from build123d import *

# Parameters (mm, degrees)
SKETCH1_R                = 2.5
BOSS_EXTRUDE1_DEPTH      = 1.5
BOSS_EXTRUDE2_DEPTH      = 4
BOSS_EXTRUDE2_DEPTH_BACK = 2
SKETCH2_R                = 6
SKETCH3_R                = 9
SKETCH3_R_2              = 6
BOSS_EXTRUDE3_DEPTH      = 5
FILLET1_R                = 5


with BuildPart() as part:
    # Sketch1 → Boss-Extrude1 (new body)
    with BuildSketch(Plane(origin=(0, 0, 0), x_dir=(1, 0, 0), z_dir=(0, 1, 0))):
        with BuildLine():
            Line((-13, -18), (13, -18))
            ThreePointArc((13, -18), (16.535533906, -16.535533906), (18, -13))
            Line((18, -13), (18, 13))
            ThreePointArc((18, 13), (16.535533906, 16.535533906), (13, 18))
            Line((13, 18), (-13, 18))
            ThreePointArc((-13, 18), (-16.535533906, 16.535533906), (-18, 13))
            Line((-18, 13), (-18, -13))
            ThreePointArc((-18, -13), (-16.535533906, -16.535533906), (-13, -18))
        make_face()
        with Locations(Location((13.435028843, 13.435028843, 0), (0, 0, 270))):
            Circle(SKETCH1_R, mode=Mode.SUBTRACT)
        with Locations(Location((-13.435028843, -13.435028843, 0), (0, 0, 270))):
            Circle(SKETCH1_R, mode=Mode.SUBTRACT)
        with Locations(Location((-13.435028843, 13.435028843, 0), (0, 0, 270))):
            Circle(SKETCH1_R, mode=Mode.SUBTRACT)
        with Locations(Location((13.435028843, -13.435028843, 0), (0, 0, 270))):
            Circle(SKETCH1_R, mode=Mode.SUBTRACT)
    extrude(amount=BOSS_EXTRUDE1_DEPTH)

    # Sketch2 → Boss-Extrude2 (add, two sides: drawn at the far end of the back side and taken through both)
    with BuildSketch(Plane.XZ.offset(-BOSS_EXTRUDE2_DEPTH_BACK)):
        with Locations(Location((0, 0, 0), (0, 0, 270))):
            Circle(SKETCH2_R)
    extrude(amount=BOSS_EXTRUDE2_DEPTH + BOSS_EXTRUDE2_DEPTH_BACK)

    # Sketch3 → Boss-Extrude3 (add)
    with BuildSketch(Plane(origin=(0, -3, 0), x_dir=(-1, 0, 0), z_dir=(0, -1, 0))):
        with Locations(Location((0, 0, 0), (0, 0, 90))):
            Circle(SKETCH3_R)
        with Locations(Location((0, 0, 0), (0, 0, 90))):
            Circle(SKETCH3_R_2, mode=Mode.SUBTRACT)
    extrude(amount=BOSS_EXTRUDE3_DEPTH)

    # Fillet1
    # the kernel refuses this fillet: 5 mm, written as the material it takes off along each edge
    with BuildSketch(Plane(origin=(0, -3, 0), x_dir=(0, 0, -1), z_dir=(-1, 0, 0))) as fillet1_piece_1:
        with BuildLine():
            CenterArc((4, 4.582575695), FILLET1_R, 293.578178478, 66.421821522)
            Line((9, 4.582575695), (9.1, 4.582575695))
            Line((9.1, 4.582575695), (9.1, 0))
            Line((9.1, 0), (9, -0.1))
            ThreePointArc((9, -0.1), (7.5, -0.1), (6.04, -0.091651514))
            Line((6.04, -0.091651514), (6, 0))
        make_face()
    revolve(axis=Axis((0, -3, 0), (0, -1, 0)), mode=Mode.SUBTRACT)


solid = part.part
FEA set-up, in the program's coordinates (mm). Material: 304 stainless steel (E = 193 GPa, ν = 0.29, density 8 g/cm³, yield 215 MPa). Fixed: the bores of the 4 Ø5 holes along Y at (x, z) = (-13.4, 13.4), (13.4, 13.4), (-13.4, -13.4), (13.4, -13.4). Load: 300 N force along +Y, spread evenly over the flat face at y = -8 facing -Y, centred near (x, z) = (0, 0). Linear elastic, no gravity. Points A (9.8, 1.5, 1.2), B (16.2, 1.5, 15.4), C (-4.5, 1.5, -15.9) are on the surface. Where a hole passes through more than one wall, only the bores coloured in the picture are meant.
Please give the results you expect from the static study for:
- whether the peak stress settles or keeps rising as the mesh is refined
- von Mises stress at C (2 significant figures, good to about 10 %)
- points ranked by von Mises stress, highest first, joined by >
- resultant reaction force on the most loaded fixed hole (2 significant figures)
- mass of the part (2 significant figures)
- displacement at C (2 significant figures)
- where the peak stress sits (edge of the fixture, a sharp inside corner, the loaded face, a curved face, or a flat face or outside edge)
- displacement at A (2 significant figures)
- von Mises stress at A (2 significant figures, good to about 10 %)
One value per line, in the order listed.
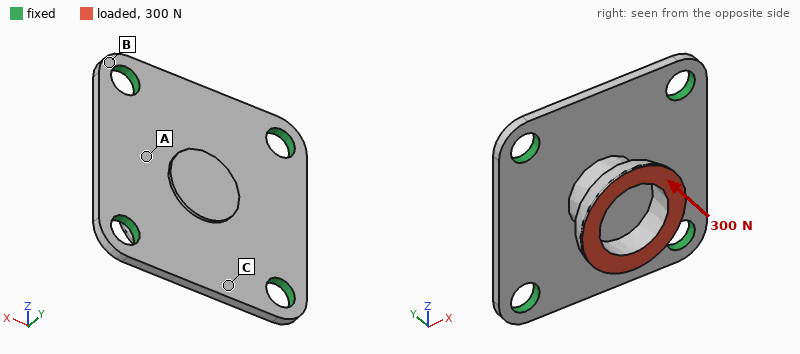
keeps rising
18 MPa
A > C > B
76 N
23 g
2.4 µm
edge of the fixture
11 µm
29 MPa
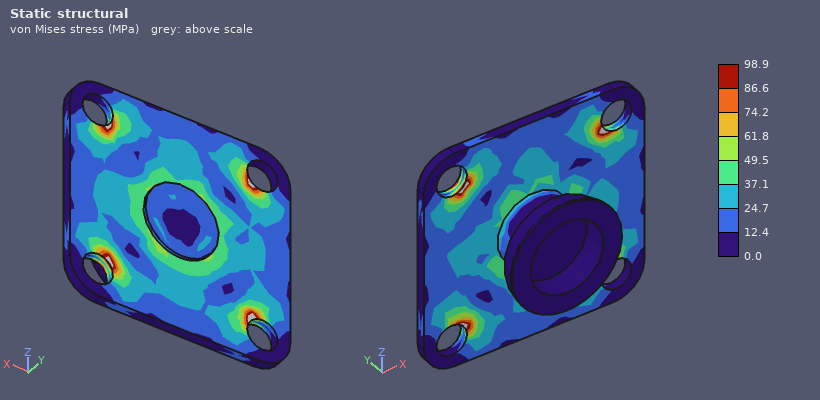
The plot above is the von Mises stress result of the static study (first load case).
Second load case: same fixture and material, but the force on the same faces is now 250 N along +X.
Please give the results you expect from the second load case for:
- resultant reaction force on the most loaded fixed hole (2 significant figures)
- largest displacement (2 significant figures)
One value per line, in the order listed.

88 N
18 µm
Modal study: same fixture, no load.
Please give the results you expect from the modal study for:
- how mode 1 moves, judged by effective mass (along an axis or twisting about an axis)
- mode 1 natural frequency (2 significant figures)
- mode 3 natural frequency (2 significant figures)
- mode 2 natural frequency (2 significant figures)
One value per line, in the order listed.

along Y
6500 Hz
9200 Hz
9100 Hz
